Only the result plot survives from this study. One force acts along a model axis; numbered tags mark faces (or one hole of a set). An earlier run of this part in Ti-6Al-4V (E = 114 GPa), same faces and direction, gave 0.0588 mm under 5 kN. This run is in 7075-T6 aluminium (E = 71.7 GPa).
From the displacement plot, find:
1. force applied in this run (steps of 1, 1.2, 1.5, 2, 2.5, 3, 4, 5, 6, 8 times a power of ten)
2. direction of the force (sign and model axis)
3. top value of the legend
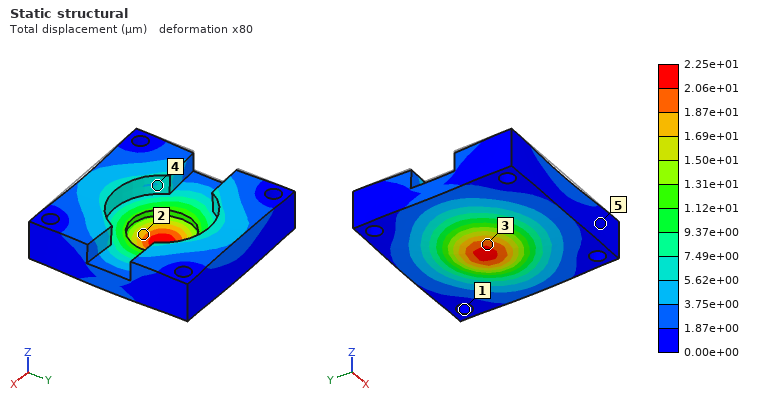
1.2 kN
-Z
2.25e+01 µm
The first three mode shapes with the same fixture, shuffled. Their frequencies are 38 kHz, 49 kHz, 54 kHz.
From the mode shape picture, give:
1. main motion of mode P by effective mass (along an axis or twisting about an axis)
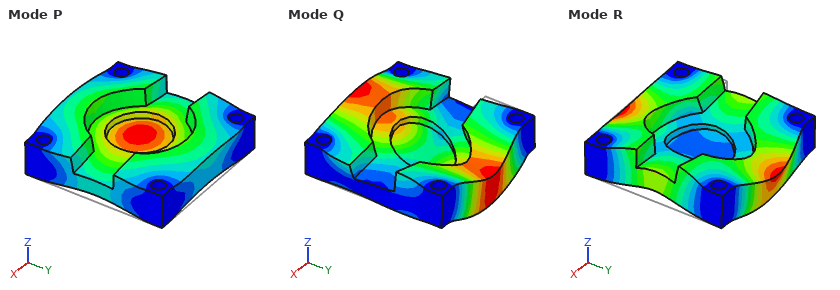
along Z
